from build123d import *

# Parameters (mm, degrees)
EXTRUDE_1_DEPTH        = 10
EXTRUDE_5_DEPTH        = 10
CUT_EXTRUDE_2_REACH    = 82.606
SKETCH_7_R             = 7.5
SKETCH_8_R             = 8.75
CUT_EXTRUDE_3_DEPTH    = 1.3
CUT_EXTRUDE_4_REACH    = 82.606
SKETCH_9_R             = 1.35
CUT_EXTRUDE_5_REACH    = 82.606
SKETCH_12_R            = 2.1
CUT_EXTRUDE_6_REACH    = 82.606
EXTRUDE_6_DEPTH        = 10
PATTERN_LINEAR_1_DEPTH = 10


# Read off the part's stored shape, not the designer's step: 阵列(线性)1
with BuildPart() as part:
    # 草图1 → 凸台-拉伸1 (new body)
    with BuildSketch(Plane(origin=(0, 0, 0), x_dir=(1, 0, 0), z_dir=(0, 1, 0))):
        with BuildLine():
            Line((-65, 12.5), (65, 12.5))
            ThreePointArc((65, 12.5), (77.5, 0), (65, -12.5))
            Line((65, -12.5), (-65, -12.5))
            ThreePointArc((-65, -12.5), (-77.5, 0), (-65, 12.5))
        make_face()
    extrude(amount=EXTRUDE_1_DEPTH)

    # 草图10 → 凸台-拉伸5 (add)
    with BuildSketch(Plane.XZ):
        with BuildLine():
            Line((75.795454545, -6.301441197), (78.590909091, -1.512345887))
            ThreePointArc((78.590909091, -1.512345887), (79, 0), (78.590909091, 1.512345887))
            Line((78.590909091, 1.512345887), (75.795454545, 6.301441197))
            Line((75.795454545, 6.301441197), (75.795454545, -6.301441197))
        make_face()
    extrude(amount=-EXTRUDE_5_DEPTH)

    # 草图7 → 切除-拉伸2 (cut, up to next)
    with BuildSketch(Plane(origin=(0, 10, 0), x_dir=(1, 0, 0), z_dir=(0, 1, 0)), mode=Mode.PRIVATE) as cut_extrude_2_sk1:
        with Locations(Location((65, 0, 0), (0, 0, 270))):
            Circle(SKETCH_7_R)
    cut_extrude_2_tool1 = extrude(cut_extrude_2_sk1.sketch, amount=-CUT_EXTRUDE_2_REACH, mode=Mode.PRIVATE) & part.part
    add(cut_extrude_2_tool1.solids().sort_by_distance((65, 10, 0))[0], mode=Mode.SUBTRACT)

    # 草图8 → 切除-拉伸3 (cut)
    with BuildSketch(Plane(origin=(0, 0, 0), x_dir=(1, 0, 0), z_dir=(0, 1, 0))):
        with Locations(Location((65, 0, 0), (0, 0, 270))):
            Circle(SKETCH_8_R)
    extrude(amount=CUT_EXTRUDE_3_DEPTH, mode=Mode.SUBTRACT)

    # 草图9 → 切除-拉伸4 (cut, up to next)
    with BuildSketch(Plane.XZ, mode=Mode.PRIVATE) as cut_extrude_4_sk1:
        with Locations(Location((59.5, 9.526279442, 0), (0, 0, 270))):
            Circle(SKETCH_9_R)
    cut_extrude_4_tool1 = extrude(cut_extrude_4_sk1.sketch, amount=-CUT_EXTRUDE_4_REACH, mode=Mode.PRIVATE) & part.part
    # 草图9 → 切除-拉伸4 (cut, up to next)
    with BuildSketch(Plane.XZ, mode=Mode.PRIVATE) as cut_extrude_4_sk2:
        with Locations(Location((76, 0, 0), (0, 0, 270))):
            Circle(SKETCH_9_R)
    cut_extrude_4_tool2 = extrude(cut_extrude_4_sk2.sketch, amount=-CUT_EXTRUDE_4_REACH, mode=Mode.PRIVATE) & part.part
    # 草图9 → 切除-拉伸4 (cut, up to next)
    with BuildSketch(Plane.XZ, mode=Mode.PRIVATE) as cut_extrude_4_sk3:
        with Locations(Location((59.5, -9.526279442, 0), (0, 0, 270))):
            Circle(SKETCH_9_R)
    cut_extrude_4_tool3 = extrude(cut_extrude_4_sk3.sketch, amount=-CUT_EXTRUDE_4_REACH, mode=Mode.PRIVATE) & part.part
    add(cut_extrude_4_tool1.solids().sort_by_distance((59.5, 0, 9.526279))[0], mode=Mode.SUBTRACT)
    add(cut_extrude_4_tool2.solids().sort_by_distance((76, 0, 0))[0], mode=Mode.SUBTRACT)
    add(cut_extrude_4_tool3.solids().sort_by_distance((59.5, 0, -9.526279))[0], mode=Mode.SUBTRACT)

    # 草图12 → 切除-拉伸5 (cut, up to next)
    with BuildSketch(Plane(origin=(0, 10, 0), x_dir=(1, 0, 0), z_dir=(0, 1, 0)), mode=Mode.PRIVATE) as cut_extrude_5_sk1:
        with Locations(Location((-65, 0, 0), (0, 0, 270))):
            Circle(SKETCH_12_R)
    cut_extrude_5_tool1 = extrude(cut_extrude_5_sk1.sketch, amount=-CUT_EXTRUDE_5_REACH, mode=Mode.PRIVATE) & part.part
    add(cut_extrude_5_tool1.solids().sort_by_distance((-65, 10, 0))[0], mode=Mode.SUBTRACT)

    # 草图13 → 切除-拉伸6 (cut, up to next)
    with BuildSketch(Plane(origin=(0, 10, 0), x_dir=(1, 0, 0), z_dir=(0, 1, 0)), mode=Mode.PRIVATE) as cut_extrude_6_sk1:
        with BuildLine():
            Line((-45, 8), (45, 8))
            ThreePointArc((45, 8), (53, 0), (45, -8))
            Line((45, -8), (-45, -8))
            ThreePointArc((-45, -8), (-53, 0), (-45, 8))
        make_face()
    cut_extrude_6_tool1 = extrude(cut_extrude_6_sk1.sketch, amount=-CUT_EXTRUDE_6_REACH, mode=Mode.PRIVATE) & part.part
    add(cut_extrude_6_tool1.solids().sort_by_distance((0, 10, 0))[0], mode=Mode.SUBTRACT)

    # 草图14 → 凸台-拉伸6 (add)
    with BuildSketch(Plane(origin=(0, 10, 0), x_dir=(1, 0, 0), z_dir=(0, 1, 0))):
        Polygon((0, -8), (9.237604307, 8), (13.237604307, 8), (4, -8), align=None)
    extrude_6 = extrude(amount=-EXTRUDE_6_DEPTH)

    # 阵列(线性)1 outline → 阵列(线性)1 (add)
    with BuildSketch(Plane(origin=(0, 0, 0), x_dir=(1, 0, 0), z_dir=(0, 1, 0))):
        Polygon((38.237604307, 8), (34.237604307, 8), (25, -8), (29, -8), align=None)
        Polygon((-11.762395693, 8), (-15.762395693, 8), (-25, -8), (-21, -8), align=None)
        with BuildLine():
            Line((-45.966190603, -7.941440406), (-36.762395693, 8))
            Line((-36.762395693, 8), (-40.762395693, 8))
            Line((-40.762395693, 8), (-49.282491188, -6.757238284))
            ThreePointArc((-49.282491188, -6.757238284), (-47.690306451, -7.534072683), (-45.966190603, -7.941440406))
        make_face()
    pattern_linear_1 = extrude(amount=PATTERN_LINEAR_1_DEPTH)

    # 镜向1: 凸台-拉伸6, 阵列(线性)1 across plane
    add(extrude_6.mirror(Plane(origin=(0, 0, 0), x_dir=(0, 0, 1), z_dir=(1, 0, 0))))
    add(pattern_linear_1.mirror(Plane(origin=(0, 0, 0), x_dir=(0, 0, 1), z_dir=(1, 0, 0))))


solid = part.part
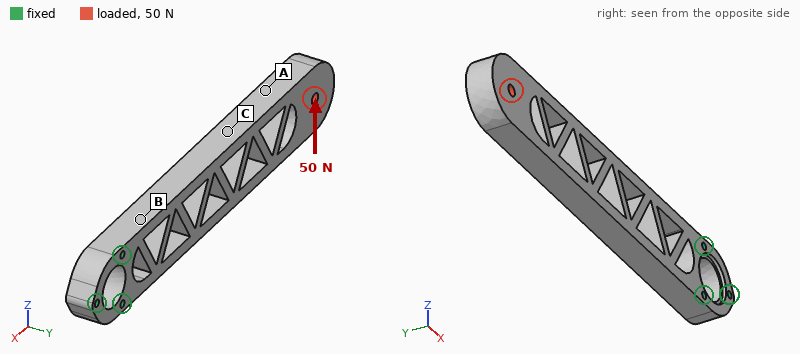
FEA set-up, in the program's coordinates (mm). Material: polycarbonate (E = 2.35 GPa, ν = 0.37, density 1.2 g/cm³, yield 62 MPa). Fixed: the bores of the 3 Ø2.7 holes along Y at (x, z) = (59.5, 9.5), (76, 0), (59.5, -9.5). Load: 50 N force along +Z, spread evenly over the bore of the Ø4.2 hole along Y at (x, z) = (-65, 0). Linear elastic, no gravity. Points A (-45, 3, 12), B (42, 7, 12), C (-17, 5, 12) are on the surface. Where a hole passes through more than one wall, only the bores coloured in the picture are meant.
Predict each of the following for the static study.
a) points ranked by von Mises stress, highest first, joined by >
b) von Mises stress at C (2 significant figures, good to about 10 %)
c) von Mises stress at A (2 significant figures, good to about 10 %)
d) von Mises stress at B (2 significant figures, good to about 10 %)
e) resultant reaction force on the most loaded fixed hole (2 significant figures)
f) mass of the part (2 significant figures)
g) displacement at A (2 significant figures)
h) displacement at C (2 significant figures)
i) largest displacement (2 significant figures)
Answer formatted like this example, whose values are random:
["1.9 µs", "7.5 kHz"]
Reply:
["B > C > A", "3.1 MPa", "1.2 MPa", "5.8 MPa", "310 N", "29 g", "1.2 mm", "0.74 mm", "1.7 mm"]
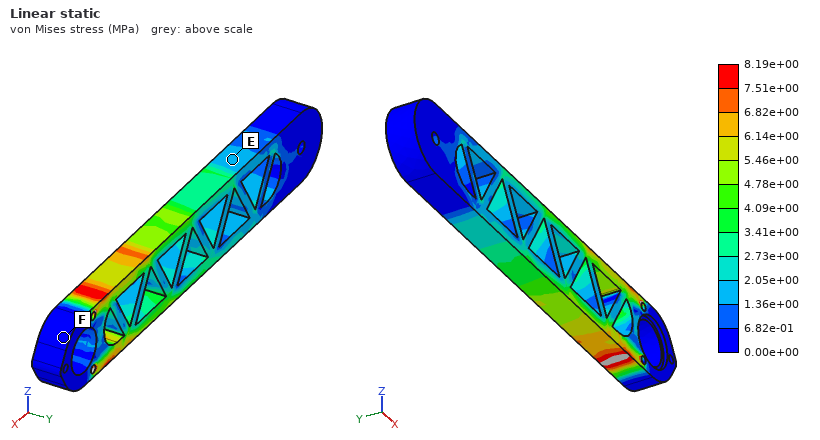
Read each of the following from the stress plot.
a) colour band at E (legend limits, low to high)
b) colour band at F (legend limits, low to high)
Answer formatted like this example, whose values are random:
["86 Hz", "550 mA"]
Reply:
["1.36e+00 to 2.05e+00 MPa", "0.00e+00 to 6.82e-01 MPa"]
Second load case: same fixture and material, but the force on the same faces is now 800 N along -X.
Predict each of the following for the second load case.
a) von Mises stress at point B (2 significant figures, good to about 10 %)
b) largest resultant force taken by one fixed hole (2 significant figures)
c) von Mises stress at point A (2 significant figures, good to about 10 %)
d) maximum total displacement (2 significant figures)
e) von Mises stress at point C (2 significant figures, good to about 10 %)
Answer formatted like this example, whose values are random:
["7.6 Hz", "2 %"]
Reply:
["6.9 MPa", "400 N", "6.4 MPa", "0.44 mm", "8.3 MPa"]
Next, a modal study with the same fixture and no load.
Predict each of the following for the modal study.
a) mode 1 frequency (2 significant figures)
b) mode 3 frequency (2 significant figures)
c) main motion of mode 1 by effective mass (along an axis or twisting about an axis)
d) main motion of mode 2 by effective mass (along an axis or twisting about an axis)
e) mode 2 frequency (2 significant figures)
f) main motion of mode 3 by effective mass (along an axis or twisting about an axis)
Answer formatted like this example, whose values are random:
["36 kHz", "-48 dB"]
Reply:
["92 Hz", "620 Hz", "along Y", "along Z", "290 Hz", "along Y"]
